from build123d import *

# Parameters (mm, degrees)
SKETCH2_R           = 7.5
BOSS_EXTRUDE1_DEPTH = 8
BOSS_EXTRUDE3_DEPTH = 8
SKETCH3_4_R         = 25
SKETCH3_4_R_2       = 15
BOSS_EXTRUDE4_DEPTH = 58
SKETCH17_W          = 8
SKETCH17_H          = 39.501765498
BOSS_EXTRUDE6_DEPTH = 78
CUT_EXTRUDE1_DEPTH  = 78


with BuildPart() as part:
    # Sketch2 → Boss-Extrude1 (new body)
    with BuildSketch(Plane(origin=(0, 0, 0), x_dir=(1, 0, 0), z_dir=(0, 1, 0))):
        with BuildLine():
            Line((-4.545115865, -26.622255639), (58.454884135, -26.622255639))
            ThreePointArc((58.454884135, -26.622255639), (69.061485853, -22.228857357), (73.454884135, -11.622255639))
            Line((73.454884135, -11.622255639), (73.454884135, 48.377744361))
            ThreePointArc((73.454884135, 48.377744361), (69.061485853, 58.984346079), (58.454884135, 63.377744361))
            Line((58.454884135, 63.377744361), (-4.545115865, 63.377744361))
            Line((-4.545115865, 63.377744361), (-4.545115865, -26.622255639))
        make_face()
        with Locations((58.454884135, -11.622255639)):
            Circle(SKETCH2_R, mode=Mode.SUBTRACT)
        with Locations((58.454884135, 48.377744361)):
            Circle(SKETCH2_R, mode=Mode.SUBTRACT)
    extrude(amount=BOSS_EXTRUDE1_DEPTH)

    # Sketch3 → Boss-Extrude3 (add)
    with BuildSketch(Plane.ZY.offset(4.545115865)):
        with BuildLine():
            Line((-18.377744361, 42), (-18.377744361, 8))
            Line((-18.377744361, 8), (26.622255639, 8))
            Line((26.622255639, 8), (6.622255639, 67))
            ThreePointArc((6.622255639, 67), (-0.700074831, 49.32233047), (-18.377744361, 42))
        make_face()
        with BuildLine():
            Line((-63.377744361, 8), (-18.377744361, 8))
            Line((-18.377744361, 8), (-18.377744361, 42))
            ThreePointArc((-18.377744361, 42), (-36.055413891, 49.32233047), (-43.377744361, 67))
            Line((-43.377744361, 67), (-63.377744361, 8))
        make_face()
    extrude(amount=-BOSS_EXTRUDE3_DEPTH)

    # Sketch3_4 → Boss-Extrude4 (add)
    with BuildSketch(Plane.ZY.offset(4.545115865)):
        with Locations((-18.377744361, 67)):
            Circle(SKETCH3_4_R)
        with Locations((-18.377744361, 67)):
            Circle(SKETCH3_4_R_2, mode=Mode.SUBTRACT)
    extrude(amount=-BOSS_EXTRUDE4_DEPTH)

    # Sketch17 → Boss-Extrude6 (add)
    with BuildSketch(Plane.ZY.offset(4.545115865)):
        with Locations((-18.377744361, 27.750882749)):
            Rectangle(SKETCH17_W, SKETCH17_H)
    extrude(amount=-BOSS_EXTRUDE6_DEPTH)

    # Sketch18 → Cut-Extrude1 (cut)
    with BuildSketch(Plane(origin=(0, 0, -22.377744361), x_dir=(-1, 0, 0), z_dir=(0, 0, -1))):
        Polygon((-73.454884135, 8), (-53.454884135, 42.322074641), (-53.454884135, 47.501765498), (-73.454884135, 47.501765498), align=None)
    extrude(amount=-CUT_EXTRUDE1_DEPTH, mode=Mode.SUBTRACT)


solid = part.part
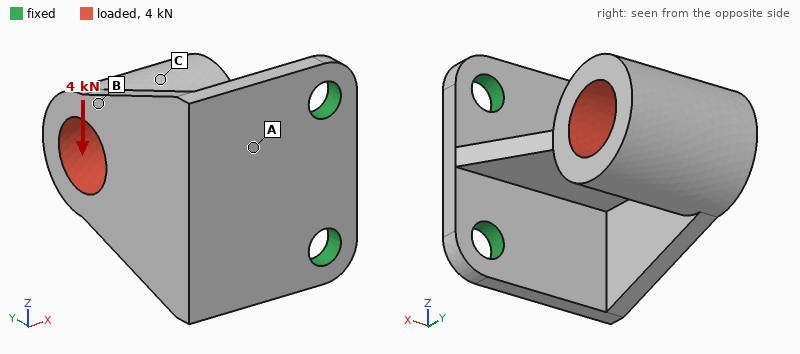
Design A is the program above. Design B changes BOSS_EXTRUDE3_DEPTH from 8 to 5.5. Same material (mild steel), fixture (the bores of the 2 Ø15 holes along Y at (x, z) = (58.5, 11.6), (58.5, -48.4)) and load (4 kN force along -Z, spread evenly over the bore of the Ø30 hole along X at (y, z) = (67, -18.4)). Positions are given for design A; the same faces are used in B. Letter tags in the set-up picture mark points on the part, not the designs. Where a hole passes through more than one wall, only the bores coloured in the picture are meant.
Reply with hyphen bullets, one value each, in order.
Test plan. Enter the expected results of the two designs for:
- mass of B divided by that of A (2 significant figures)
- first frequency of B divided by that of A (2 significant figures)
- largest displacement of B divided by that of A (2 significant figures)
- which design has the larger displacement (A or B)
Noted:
- 0.96
- 1.0
- 1.2
- B
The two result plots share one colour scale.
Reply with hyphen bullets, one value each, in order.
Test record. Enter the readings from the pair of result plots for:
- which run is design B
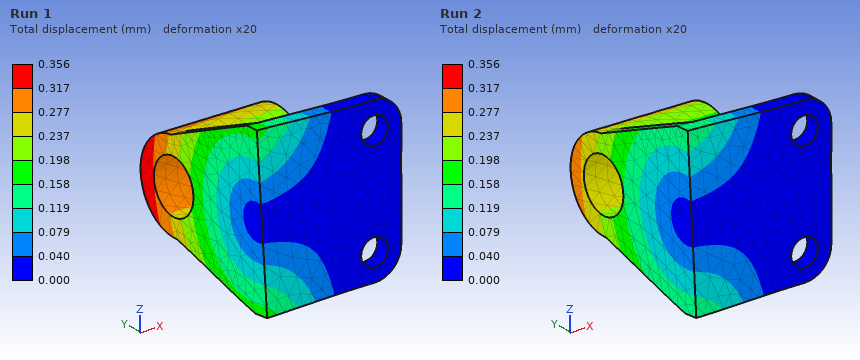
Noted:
- Run 1
